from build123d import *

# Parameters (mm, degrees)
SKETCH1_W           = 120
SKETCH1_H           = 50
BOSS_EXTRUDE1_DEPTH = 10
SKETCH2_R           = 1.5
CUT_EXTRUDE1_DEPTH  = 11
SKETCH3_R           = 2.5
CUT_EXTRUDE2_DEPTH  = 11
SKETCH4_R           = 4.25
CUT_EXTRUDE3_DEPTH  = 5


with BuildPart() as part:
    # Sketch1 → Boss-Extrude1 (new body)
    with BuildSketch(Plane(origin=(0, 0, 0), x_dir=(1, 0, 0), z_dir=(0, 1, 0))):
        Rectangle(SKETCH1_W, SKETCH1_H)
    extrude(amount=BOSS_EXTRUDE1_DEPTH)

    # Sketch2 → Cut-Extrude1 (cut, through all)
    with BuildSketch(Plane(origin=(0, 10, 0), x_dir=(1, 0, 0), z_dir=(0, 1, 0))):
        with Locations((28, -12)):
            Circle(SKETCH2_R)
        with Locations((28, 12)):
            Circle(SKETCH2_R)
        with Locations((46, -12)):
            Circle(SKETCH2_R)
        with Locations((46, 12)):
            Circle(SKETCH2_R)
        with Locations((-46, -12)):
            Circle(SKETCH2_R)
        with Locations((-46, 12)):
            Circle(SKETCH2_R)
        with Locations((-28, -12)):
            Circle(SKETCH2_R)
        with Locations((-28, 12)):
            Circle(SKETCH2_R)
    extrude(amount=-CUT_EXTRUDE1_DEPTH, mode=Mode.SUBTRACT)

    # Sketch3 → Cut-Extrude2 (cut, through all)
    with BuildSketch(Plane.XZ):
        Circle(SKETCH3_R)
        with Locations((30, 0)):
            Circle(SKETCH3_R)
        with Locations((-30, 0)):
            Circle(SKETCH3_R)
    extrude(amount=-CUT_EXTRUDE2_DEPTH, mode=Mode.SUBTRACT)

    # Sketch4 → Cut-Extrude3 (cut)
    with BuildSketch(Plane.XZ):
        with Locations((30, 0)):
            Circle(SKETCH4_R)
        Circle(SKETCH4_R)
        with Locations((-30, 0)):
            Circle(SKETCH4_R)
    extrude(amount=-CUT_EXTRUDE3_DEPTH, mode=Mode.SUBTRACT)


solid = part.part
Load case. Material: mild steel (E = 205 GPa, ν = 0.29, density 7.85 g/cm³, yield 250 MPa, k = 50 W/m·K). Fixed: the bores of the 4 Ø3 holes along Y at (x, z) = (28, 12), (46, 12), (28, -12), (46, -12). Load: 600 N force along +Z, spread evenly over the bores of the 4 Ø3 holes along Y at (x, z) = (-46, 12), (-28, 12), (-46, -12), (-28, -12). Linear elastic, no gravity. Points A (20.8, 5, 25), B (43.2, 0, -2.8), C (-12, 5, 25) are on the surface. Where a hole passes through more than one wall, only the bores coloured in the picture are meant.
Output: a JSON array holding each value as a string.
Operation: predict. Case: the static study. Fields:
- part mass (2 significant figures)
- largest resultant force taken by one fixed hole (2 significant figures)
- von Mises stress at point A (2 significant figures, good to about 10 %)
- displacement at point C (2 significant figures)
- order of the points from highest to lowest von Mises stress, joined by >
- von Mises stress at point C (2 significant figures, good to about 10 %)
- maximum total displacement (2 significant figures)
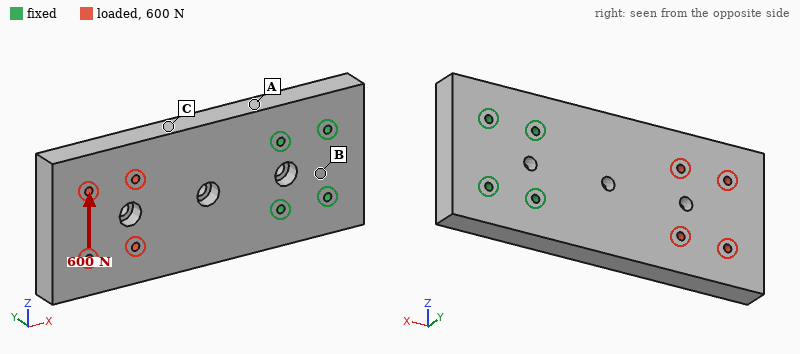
["460 g", "1.0 kN", "7.1 MPa", "3.3 µm", "A > C > B", "3.5 MPa", "7.2 µm"]
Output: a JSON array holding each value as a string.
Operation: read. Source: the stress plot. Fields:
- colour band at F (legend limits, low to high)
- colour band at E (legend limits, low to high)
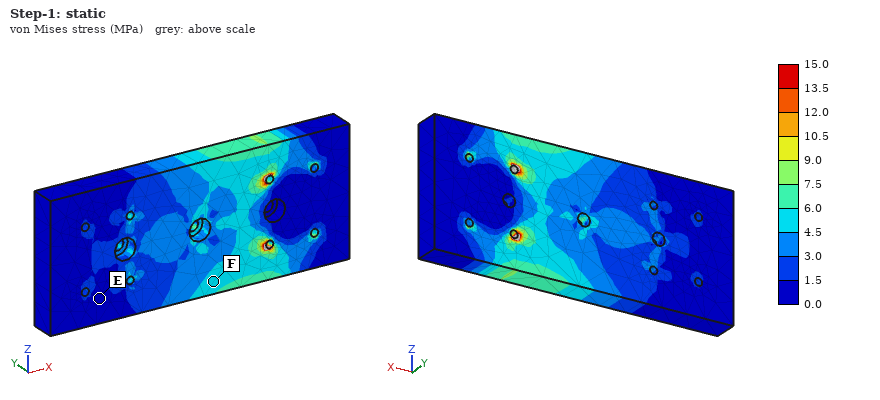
["4.5 to 6.0 MPa", "0.0 to 1.5 MPa"]
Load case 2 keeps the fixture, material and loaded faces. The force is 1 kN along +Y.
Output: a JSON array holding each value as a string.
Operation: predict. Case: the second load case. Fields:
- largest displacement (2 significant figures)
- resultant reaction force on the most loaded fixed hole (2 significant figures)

["0.19 mm", "1.2 kN"]
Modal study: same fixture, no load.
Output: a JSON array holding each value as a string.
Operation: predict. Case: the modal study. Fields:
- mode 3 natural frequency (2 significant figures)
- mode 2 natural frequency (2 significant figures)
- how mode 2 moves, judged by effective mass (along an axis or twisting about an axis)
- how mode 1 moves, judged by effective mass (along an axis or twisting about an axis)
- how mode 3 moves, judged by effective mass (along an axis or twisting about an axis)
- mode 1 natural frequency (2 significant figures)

["3800 Hz", "3500 Hz", "twisting about X", "along Y", "along Z", "1000 Hz"]
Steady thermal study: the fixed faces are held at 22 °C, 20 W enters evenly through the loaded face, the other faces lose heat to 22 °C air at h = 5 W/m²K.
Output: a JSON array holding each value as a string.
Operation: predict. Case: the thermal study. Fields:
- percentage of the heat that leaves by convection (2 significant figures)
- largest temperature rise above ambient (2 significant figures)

["9.8 %", "55 K"]
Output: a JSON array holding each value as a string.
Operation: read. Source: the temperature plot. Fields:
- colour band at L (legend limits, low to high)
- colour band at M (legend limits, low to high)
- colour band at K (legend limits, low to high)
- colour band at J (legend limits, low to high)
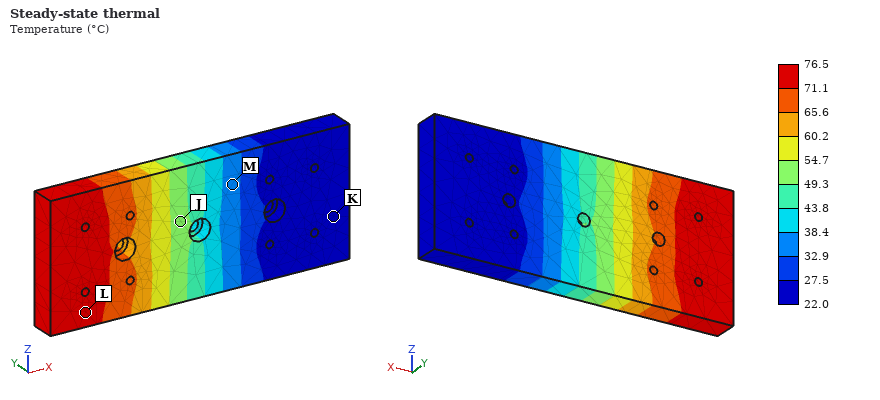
["71.1 to 76.5 °C", "32.9 to 38.4 °C", "22.0 to 27.5 °C", "49.3 to 54.7 °C"]
